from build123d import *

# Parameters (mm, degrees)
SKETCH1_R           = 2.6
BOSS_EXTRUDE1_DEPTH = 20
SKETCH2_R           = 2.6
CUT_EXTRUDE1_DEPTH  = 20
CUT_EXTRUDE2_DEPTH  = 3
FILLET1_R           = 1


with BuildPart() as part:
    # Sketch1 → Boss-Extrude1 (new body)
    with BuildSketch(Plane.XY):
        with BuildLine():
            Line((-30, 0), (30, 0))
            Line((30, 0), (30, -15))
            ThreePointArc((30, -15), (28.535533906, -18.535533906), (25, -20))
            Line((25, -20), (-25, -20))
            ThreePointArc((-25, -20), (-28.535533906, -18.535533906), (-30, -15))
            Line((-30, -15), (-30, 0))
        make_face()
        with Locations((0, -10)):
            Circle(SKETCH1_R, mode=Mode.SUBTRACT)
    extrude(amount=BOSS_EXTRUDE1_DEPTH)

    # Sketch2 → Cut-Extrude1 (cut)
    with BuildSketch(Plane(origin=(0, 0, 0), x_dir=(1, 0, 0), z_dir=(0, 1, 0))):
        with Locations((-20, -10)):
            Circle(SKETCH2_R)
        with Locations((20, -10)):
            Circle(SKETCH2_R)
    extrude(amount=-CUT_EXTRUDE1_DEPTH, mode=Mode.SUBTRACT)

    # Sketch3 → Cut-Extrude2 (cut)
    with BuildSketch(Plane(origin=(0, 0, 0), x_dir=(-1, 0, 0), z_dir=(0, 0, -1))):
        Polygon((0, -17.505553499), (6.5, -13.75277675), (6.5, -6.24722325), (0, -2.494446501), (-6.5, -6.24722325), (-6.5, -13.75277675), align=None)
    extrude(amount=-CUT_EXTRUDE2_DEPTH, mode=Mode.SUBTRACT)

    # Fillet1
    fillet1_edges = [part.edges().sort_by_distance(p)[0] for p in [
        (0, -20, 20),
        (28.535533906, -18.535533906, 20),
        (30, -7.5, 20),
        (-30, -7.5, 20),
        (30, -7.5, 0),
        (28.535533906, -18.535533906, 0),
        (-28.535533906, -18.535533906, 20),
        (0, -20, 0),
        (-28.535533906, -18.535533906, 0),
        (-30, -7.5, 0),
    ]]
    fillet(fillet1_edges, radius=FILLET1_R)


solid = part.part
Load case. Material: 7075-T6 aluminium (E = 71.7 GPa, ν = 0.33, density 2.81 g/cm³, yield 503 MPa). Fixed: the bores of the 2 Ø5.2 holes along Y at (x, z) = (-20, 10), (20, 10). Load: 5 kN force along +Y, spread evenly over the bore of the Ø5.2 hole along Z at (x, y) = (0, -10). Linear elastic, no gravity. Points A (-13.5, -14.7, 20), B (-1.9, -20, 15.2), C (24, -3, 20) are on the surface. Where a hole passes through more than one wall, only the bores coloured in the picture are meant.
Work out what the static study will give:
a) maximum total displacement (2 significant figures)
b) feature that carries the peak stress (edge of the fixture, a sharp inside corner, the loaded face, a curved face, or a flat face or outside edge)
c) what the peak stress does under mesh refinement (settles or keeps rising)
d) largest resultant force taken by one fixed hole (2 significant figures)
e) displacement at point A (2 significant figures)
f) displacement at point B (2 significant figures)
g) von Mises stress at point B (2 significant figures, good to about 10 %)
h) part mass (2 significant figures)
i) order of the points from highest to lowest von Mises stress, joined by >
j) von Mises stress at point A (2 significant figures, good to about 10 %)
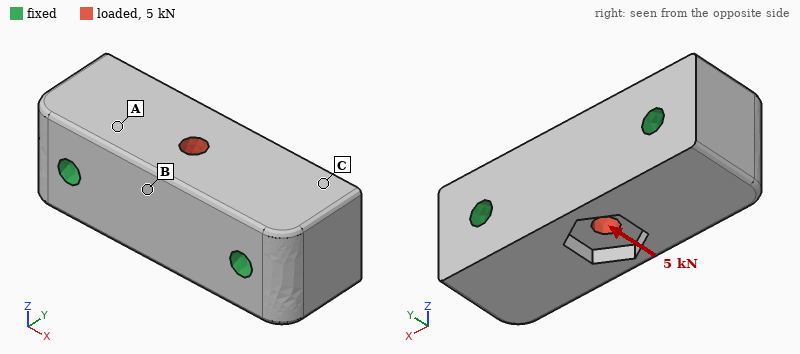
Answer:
8.6 µm
edge of the fixture
keeps rising
2.5 kN
2.9 µm
6.9 µm
22 MPa
62 g
B > A > C
13 MPa
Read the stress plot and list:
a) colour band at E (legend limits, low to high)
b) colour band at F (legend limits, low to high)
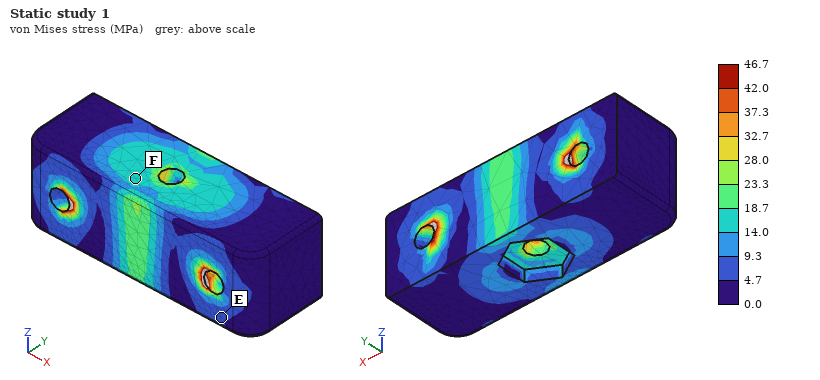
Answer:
4.7 to 9.3 MPa
14.0 to 18.7 MPa
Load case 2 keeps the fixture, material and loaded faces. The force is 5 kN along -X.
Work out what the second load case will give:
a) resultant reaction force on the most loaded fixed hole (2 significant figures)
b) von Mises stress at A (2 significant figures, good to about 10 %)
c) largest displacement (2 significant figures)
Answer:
2.5 kN
4.9 MPa
2.9 µm
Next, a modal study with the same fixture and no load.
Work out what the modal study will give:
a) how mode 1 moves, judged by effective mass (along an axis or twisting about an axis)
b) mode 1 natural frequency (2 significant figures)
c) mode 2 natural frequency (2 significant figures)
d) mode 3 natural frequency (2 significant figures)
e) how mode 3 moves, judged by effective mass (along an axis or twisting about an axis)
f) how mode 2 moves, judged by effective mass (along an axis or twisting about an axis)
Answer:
along Z
26 kHz
32 kHz
36 kHz
twisting about X
along Y
